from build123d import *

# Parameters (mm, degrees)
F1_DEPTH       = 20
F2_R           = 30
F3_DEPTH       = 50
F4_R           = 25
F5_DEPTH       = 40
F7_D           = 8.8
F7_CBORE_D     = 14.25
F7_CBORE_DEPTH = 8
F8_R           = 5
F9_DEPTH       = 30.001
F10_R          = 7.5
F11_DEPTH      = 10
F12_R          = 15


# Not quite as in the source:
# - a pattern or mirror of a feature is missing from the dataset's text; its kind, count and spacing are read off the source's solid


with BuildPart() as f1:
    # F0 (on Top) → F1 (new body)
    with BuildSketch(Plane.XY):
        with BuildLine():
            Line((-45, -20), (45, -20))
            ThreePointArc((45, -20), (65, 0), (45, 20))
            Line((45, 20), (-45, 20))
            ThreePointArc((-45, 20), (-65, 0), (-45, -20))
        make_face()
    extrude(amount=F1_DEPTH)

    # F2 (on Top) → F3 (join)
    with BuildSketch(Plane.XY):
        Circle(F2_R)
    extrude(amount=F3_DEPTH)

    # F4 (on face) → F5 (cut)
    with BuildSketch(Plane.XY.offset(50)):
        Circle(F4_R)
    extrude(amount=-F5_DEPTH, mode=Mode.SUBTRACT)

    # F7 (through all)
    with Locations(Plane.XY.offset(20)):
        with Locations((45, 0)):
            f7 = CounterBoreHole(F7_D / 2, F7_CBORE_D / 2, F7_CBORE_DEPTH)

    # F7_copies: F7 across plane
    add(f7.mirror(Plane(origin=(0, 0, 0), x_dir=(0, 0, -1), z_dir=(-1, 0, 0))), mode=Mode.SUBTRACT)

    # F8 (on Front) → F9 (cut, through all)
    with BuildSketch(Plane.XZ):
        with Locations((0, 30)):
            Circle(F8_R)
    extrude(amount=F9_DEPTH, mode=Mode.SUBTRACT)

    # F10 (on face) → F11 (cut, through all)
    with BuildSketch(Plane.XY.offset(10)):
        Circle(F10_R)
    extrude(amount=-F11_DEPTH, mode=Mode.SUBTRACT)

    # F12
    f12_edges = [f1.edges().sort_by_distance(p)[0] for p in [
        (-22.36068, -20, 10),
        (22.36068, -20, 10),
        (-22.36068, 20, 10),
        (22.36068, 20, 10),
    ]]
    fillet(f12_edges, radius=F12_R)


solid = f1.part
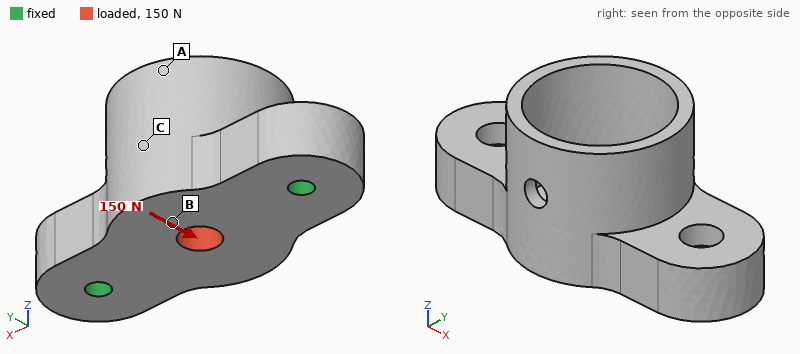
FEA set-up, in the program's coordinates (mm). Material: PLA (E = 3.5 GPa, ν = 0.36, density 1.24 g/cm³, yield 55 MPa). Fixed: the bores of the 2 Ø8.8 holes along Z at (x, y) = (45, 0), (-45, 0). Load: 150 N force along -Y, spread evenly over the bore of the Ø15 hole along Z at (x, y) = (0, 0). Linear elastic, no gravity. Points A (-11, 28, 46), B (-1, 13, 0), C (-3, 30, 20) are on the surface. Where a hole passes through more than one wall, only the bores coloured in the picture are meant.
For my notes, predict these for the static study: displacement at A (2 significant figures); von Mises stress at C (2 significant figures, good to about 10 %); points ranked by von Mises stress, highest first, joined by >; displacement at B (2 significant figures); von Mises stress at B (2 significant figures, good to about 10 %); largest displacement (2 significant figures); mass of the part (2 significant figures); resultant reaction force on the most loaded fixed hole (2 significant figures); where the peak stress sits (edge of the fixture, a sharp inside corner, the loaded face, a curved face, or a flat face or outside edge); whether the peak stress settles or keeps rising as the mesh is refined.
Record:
1.8 µm
0.18 MPa
B > C > A
7.5 µm
0.35 MPa
8.0 µm
140 g
75 N
edge of the fixture
keeps rising
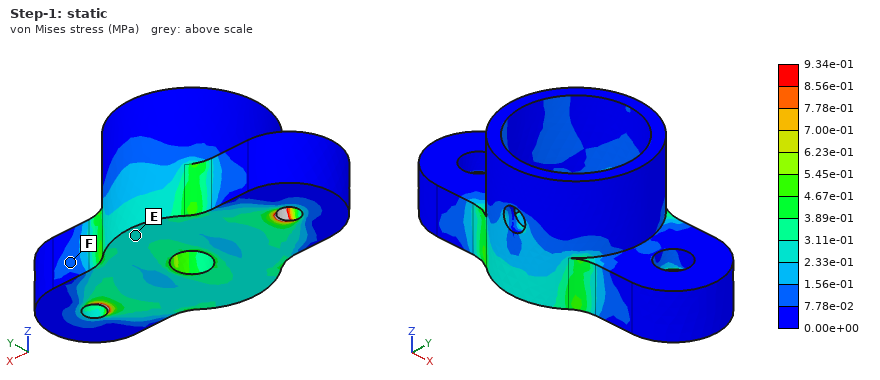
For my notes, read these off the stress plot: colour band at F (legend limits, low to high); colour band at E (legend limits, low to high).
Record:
7.78e-02 to 1.56e-01 MPa
2.33e-01 to 3.11e-01 MPa
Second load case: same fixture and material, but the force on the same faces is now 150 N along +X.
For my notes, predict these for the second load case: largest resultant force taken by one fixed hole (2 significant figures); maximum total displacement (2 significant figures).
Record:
75 N
2.8 µm
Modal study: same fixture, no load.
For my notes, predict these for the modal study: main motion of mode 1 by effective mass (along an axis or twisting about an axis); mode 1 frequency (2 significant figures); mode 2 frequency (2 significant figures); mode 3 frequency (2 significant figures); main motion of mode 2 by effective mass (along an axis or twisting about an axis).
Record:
along Y
1400 Hz
1700 Hz
2300 Hz
along Z
